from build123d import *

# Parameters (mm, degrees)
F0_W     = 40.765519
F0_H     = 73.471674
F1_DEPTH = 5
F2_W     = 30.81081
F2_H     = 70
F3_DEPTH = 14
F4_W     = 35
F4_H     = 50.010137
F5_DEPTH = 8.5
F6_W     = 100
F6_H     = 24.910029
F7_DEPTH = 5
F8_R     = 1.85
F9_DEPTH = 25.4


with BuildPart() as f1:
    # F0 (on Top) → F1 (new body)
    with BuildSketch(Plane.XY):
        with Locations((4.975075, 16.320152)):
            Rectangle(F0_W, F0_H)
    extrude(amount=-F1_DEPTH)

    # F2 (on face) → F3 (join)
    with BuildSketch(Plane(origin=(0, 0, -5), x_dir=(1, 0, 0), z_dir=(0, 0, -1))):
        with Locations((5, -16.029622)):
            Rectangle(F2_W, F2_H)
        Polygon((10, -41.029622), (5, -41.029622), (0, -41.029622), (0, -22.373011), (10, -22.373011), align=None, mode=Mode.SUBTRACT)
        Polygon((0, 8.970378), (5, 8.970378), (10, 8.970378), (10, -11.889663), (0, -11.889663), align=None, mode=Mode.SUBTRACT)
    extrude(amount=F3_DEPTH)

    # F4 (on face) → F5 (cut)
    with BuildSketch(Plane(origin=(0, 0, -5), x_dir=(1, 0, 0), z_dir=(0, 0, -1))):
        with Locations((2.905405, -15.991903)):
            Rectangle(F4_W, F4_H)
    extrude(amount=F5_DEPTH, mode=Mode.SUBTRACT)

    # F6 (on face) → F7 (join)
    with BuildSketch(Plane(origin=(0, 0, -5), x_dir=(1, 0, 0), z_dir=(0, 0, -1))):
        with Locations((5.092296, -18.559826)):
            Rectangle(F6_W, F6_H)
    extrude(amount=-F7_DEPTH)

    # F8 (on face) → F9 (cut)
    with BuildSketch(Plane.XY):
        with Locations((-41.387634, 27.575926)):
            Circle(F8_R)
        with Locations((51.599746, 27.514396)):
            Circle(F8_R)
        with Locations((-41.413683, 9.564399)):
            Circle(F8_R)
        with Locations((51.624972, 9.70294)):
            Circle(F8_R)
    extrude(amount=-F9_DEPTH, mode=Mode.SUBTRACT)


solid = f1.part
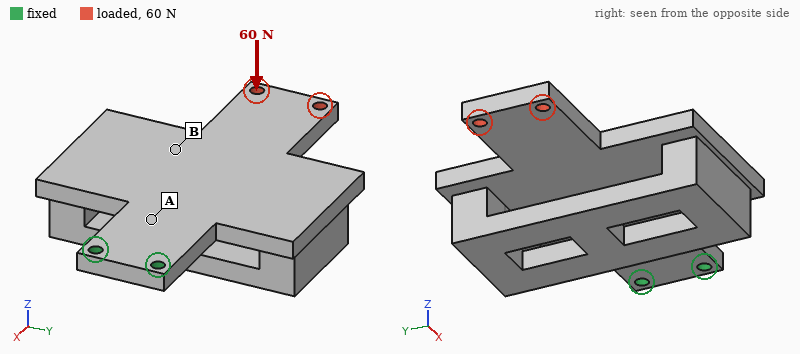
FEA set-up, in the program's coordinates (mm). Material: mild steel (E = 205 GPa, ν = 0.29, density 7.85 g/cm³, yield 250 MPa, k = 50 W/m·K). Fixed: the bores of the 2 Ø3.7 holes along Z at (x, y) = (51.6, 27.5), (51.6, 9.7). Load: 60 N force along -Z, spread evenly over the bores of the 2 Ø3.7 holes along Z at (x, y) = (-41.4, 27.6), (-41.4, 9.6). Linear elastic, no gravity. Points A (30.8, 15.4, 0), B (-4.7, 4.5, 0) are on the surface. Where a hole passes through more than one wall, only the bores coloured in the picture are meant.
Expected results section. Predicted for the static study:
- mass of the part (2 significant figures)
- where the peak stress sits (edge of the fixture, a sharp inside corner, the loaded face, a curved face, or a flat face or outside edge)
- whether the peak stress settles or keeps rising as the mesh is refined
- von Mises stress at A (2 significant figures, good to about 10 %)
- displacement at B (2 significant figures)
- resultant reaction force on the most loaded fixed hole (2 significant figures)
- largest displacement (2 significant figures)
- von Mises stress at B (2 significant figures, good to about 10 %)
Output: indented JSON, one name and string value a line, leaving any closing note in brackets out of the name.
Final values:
{
  "mass of the part": "290 g",
  "where the peak stress sits": "edge of the fixture",
  "whether the peak stress settles or keeps rising as the mesh is refined": "keeps rising",
  "von Mises stress at A": "40 MPa",
  "displacement at B": "0.12 mm",
  "resultant reaction force on the most loaded fixed hole": "30 N",
  "largest displacement": "0.27 mm",
  "von Mises stress at B": "7.7 MPa"
}
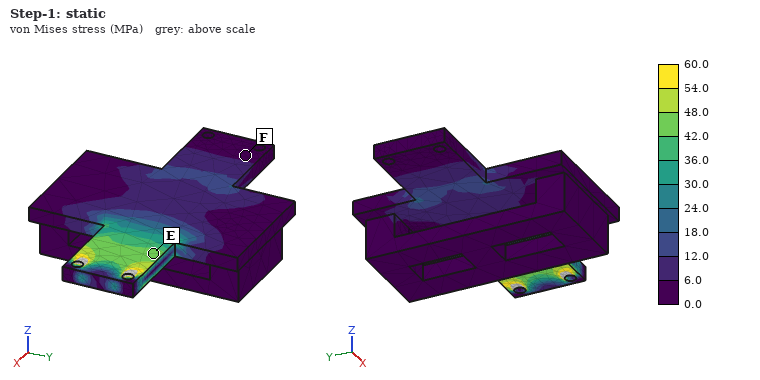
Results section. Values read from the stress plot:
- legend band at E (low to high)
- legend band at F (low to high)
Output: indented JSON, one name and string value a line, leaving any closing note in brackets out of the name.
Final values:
{
  "legend band at E": "42.0 to 48.0 MPa",
  "legend band at F": "0.0 to 6.0 MPa"
}
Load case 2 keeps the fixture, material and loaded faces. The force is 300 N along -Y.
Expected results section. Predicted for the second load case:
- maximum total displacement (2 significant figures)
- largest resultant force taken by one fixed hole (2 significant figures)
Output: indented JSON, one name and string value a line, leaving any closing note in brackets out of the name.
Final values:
{
  "maximum total displacement": "54 µm",
  "largest resultant force taken by one fixed hole": "1.5 kN"
}
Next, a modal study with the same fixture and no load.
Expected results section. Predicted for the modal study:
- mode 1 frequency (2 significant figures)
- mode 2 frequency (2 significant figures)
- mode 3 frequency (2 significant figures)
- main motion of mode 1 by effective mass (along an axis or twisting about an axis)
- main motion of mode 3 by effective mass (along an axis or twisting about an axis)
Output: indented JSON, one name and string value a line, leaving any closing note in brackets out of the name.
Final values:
{
  "mode 1 frequency": "320 Hz",
  "mode 2 frequency": "700 Hz",
  "mode 3 frequency": "1400 Hz",
  "main motion of mode 1 by effective mass": "along Z",
  "main motion of mode 3 by effective mass": "along Y"
}
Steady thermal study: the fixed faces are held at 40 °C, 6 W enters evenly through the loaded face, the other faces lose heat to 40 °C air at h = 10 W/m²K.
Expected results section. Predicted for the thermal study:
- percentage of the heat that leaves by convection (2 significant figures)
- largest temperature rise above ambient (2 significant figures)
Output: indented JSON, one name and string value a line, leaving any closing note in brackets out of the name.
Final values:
{
  "percentage of the heat that leaves by convection": "52 %",
  "largest temperature rise above ambient": "56 K"
}
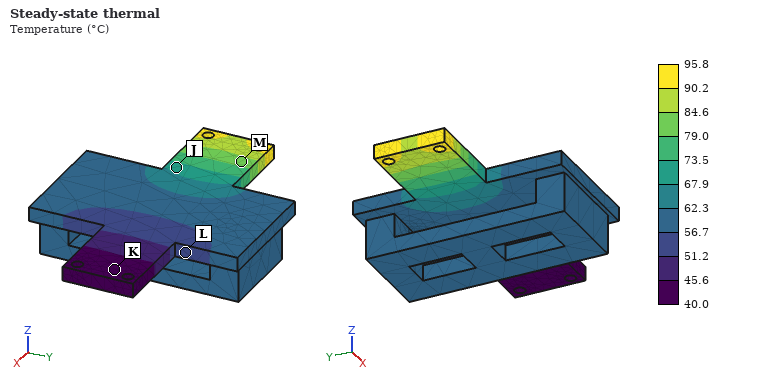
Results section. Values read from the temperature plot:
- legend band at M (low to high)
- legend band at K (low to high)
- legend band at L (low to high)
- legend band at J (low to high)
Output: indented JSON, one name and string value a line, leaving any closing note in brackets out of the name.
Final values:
{
  "legend band at M": "79.0 to 84.6 °C",
  "legend band at K": "40.0 to 45.6 °C",
  "legend band at L": "51.2 to 56.7 °C",
  "legend band at J": "67.9 to 73.5 °C"
}
